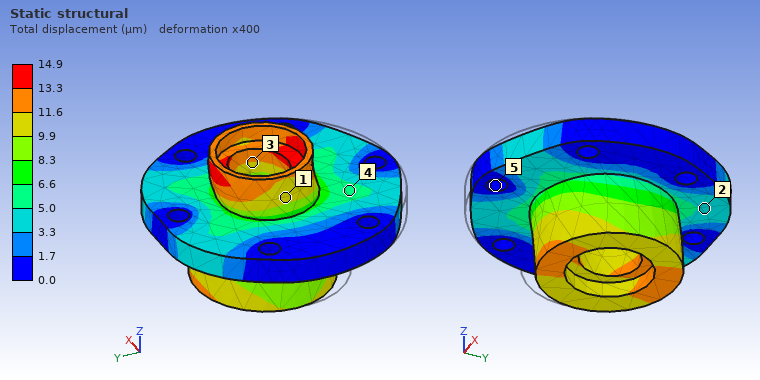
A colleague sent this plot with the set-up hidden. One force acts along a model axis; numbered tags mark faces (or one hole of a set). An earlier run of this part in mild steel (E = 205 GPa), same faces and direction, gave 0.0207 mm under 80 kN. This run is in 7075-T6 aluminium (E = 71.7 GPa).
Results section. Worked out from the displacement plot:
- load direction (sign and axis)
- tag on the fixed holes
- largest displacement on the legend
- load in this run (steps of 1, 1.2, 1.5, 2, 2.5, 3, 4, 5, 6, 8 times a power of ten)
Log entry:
+Y
5
14.9 µm
20 kN
